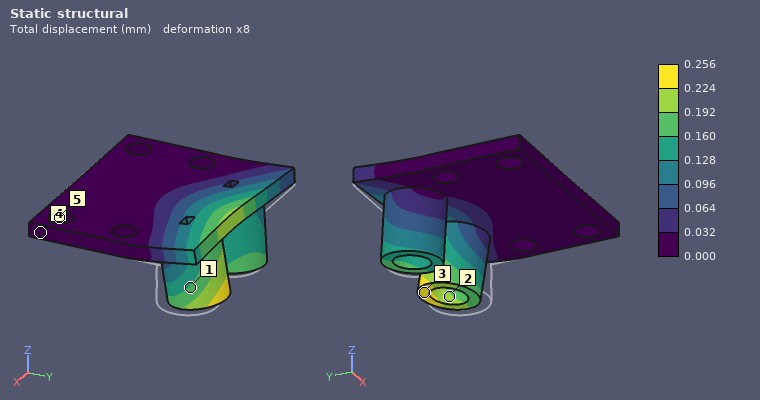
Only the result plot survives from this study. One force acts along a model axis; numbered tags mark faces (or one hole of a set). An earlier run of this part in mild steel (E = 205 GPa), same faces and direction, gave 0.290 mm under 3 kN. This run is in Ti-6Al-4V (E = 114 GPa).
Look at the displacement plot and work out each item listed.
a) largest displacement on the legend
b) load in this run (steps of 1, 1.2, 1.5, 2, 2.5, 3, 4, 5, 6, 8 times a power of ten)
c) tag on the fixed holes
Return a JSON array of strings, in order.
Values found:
["0.256 mm", "1.5 kN", "5"]
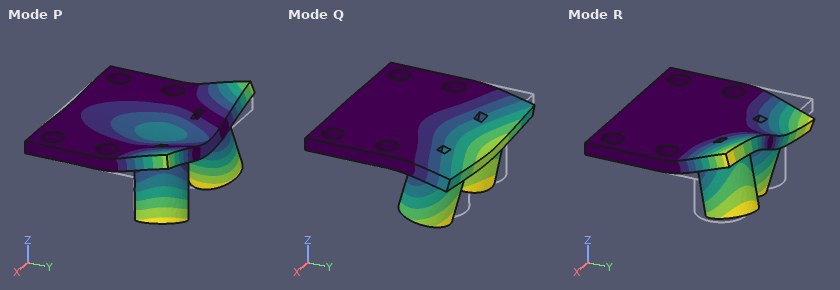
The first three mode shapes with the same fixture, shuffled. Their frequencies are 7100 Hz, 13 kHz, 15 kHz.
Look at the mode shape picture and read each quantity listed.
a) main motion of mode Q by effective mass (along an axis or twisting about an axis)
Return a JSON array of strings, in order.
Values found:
["along Z"]
